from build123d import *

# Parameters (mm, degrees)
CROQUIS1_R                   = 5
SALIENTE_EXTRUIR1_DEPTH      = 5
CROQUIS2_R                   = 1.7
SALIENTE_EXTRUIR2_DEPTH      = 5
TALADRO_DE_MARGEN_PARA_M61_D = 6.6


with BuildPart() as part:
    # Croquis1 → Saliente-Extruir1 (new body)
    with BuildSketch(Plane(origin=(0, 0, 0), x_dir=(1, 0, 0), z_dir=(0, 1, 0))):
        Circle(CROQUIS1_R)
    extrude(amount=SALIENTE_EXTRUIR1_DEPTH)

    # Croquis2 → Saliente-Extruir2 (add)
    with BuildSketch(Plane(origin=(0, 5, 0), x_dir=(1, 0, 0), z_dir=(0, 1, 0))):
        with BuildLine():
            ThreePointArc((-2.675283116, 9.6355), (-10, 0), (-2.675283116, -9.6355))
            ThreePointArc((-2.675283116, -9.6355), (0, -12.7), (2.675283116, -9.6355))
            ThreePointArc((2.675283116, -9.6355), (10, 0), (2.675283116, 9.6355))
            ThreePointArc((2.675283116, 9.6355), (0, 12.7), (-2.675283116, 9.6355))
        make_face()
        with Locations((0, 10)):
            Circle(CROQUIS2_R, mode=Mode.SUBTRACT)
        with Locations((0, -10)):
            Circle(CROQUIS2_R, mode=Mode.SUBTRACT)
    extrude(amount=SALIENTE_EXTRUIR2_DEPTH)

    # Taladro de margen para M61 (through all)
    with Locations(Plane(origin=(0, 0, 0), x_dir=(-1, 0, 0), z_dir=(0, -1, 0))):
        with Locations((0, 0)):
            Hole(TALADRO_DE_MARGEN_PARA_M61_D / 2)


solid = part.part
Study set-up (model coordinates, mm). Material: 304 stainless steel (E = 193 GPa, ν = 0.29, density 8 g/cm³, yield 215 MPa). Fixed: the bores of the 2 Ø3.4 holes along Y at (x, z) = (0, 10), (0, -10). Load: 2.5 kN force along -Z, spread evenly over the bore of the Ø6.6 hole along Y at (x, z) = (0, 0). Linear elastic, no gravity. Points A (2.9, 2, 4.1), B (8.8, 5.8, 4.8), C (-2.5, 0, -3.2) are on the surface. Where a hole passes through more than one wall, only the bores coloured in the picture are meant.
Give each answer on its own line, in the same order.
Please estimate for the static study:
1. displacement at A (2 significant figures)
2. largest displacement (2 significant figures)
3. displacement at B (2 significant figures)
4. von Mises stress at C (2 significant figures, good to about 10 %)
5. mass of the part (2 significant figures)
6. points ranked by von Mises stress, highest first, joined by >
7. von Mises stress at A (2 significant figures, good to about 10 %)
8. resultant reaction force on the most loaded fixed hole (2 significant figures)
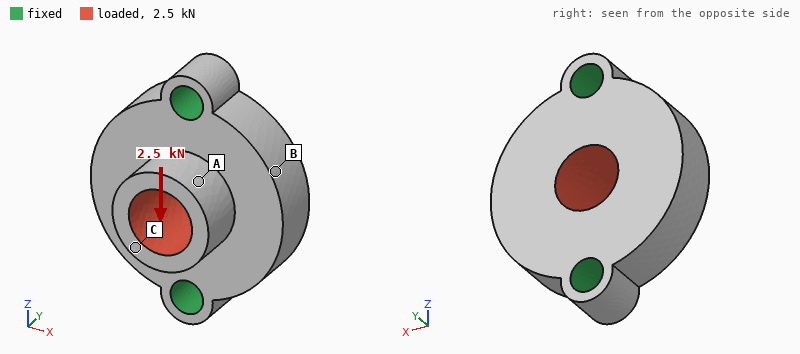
3.7 µm
5.0 µm
1.2 µm
35 MPa
13 g
C > A > B
20 MPa
1.3 kN
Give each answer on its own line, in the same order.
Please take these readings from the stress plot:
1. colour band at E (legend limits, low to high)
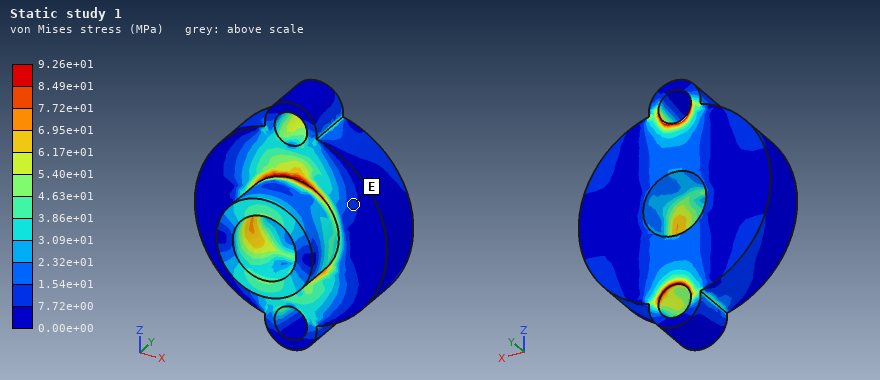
7.72e+00 to 1.54e+01 MPa
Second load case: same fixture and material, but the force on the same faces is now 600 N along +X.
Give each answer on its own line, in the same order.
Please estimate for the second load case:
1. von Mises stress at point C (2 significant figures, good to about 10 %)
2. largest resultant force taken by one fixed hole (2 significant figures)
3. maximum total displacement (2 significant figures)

6.2 MPa
300 N
2.6 µm
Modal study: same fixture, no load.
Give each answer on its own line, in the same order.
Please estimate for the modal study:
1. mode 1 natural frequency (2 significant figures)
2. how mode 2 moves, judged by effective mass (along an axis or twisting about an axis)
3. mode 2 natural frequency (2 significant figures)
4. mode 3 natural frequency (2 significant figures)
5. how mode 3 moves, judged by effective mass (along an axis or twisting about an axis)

25 kHz
along Y
34 kHz
58 kHz
along X
